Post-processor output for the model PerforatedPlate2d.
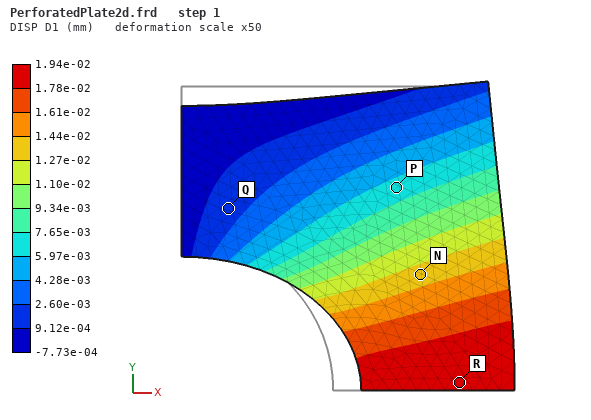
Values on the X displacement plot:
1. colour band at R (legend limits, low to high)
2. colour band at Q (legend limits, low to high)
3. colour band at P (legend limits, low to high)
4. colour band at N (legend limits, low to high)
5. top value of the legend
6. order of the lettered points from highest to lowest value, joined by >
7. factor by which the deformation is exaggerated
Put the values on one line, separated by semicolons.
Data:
1.78e-02 to 1.94e-02 mm; 9.12e-04 to 2.60e-03 mm; 5.97e-03 to 7.65e-03 mm; 1.27e-02 to 1.44e-02 mm; 1.94e-02 mm; R > N > P > Q; 50
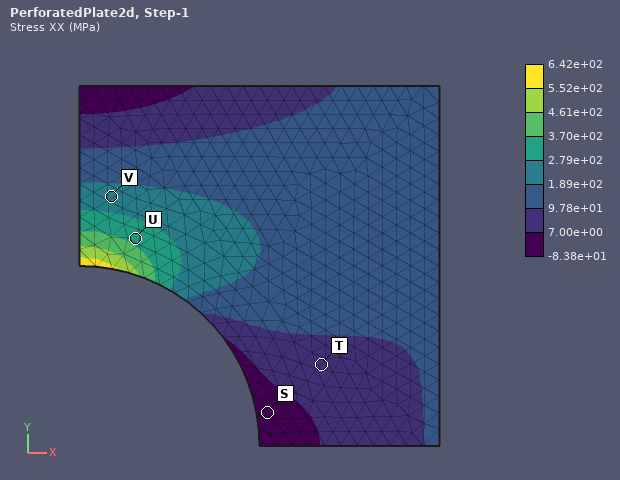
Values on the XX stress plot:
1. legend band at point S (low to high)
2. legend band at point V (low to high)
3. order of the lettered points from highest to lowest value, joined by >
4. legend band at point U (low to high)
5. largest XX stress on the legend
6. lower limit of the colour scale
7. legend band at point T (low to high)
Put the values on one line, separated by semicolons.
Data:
-8.38e+01 to 7.00e+00 MPa; 1.89e+02 to 2.79e+02 MPa; U > V > T > S; 2.79e+02 to 3.70e+02 MPa; 6.42e+02 MPa; -8.38e+01 MPa; 7.00e+00 to 9.78e+01 MPa
